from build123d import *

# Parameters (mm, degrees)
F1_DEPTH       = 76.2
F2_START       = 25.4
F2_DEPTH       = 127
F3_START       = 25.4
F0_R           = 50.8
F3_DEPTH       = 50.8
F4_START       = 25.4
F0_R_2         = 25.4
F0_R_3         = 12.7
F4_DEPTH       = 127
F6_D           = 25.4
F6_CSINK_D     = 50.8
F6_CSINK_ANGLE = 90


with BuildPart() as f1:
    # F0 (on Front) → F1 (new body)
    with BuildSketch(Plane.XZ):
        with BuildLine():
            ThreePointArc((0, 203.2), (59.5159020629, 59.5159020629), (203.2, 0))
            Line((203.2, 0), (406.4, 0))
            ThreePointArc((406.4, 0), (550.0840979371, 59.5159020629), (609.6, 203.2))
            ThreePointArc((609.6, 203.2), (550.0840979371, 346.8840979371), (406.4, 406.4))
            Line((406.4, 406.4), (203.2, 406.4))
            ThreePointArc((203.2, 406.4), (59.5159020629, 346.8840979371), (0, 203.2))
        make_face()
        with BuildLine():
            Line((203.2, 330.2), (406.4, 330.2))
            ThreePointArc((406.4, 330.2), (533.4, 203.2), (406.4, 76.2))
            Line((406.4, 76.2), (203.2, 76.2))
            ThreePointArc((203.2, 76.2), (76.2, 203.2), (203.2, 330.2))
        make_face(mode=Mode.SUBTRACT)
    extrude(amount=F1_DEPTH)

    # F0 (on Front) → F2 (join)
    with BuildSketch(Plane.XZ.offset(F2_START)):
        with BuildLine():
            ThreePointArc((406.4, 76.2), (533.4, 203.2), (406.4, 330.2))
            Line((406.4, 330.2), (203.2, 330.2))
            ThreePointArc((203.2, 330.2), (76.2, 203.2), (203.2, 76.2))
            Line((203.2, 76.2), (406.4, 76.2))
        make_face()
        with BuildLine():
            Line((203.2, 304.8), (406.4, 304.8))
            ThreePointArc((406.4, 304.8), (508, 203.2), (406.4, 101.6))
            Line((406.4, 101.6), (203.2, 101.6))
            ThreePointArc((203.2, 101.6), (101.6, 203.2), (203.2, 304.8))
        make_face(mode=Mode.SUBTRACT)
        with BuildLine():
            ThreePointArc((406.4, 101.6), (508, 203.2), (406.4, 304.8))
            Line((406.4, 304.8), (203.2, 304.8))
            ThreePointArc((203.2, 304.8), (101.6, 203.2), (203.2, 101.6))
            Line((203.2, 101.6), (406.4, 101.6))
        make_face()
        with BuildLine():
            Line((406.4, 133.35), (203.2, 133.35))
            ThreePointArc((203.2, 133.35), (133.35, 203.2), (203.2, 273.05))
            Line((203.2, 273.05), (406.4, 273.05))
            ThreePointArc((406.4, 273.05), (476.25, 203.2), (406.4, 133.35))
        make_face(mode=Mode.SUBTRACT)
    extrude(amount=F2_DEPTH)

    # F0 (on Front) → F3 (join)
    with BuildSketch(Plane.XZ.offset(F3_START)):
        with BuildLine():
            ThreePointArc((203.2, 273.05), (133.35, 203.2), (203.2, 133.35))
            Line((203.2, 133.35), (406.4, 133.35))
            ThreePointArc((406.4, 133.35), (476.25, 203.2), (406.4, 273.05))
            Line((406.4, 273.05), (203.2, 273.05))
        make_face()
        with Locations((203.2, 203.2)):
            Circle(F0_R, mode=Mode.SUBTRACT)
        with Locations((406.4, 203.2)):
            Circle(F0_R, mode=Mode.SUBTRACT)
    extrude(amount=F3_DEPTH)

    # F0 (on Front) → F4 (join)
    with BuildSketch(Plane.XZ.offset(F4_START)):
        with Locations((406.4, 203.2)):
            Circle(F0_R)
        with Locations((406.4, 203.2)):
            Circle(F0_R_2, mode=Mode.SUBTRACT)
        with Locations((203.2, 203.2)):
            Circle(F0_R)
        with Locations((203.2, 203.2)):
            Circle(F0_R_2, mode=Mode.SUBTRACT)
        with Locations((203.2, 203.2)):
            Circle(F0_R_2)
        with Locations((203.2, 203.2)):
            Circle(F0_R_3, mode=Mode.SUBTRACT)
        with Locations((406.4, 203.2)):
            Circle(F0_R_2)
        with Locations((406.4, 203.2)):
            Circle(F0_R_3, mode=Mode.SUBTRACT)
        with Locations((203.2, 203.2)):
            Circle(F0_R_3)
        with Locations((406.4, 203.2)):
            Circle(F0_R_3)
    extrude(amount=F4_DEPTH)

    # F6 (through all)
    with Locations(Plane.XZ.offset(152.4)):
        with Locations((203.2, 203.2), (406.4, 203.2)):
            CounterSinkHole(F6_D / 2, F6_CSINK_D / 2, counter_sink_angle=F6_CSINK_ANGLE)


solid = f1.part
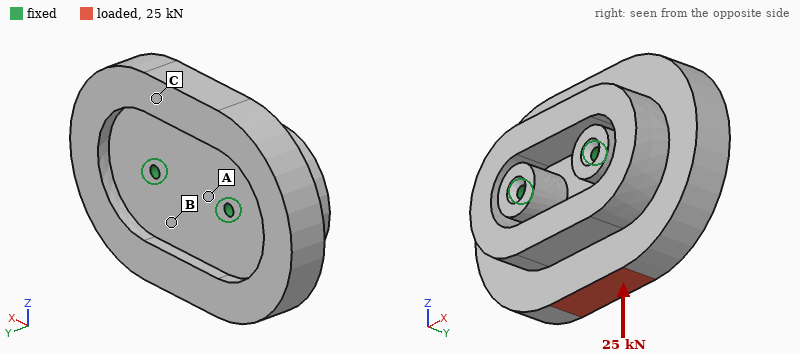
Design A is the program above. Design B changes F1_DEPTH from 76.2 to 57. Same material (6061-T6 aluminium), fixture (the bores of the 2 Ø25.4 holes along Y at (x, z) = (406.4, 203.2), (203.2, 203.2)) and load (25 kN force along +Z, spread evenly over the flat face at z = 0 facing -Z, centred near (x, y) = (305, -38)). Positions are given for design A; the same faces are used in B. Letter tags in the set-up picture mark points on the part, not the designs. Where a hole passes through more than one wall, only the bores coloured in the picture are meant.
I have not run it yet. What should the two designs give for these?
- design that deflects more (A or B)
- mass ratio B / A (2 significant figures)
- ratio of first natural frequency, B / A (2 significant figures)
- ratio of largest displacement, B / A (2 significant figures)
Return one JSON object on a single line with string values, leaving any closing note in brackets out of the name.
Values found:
{"design that deflects more": "B", "mass ratio B / A": "0.89", "ratio of first natural frequency, B / A": "1.1", "ratio of largest displacement, B / A": "1.7"}
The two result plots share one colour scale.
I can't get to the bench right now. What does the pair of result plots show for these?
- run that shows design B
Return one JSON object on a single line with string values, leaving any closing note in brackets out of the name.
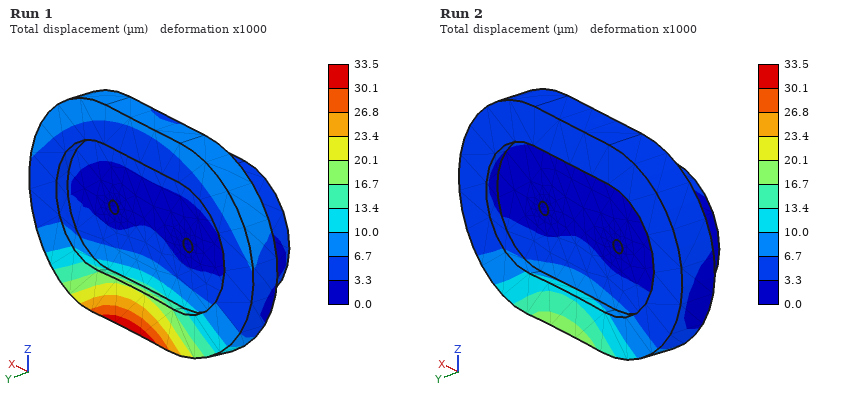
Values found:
{"run that shows design B": "Run 1"}
